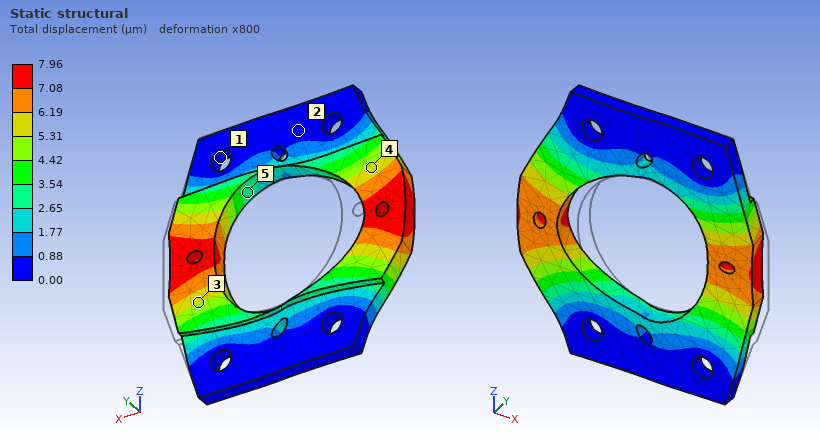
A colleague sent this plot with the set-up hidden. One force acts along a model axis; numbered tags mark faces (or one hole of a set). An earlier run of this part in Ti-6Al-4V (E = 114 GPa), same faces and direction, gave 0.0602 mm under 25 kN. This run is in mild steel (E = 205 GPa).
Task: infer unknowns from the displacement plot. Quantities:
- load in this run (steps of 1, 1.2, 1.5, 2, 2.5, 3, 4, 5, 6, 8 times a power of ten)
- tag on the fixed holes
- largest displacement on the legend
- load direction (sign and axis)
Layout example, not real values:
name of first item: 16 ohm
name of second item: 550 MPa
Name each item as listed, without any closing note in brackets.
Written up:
load in this run: 6 kN
tag on the fixed holes: 1
largest displacement on the legend: 7.96 µm
load direction: -X
